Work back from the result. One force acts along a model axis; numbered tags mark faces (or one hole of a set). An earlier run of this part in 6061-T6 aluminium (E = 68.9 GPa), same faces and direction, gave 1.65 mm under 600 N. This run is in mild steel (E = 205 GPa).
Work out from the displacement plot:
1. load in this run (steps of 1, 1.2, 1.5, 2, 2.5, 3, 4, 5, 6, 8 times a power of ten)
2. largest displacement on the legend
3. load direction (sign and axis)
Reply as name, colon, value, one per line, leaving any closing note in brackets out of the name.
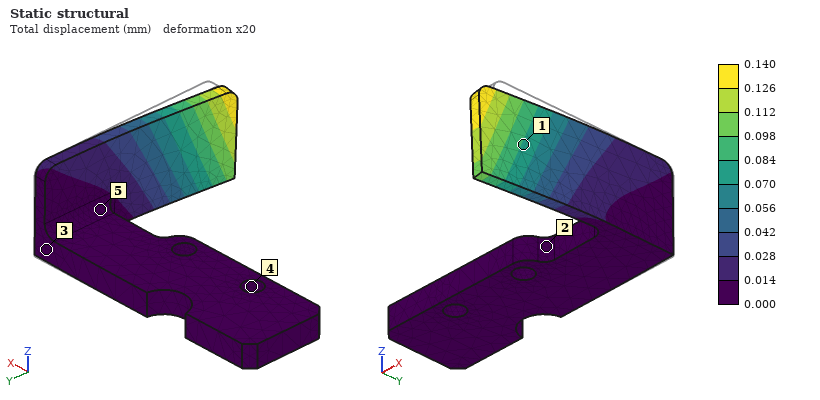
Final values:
load in this run: 150 N
largest displacement on the legend: 0.140 mm
load direction: -X
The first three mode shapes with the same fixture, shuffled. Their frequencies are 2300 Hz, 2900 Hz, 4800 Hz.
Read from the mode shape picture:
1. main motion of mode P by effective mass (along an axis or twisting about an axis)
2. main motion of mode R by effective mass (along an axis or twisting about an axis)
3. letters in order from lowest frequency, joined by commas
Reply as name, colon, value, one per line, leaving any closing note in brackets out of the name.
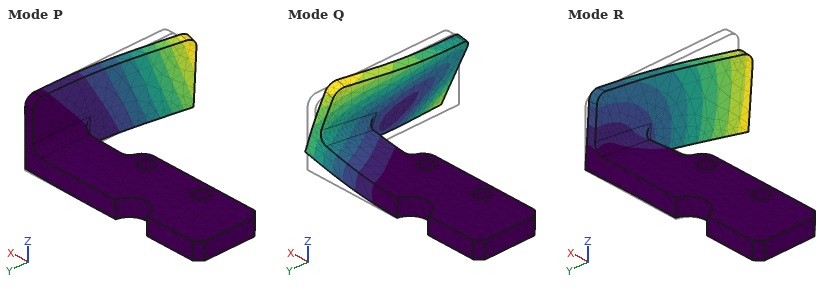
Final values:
main motion of mode P by effective mass: along X
main motion of mode R by effective mass: along Z
letters in order from lowest frequency, joined by commas: P, R, Q
